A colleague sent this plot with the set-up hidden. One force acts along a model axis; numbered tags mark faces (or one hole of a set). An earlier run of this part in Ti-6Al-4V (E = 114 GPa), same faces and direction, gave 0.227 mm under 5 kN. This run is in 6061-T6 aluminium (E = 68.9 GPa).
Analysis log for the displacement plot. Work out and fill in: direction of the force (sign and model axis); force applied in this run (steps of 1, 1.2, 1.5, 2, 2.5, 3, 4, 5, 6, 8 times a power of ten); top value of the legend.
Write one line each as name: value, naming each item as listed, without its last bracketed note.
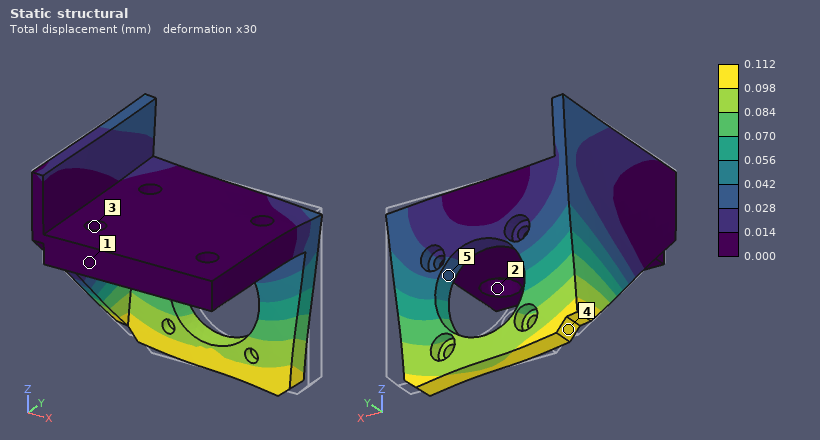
direction of the force: -X
force applied in this run: 1.5 kN
top value of the legend: 0.112 mm
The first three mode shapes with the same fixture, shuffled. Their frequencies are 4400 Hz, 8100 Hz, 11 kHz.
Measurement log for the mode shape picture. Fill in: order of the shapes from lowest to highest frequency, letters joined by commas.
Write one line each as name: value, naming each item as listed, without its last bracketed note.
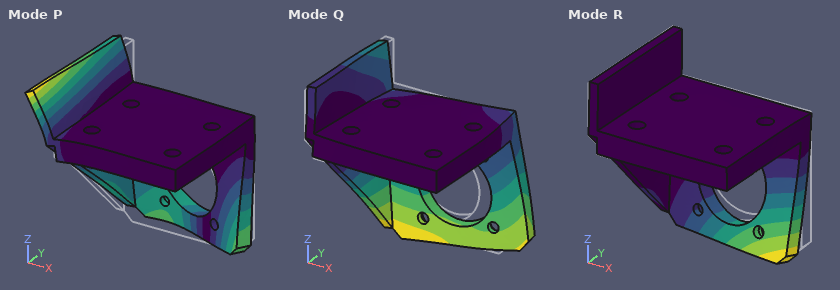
order of the shapes from lowest to highest frequency, letters joined by commas: R, Q, P
